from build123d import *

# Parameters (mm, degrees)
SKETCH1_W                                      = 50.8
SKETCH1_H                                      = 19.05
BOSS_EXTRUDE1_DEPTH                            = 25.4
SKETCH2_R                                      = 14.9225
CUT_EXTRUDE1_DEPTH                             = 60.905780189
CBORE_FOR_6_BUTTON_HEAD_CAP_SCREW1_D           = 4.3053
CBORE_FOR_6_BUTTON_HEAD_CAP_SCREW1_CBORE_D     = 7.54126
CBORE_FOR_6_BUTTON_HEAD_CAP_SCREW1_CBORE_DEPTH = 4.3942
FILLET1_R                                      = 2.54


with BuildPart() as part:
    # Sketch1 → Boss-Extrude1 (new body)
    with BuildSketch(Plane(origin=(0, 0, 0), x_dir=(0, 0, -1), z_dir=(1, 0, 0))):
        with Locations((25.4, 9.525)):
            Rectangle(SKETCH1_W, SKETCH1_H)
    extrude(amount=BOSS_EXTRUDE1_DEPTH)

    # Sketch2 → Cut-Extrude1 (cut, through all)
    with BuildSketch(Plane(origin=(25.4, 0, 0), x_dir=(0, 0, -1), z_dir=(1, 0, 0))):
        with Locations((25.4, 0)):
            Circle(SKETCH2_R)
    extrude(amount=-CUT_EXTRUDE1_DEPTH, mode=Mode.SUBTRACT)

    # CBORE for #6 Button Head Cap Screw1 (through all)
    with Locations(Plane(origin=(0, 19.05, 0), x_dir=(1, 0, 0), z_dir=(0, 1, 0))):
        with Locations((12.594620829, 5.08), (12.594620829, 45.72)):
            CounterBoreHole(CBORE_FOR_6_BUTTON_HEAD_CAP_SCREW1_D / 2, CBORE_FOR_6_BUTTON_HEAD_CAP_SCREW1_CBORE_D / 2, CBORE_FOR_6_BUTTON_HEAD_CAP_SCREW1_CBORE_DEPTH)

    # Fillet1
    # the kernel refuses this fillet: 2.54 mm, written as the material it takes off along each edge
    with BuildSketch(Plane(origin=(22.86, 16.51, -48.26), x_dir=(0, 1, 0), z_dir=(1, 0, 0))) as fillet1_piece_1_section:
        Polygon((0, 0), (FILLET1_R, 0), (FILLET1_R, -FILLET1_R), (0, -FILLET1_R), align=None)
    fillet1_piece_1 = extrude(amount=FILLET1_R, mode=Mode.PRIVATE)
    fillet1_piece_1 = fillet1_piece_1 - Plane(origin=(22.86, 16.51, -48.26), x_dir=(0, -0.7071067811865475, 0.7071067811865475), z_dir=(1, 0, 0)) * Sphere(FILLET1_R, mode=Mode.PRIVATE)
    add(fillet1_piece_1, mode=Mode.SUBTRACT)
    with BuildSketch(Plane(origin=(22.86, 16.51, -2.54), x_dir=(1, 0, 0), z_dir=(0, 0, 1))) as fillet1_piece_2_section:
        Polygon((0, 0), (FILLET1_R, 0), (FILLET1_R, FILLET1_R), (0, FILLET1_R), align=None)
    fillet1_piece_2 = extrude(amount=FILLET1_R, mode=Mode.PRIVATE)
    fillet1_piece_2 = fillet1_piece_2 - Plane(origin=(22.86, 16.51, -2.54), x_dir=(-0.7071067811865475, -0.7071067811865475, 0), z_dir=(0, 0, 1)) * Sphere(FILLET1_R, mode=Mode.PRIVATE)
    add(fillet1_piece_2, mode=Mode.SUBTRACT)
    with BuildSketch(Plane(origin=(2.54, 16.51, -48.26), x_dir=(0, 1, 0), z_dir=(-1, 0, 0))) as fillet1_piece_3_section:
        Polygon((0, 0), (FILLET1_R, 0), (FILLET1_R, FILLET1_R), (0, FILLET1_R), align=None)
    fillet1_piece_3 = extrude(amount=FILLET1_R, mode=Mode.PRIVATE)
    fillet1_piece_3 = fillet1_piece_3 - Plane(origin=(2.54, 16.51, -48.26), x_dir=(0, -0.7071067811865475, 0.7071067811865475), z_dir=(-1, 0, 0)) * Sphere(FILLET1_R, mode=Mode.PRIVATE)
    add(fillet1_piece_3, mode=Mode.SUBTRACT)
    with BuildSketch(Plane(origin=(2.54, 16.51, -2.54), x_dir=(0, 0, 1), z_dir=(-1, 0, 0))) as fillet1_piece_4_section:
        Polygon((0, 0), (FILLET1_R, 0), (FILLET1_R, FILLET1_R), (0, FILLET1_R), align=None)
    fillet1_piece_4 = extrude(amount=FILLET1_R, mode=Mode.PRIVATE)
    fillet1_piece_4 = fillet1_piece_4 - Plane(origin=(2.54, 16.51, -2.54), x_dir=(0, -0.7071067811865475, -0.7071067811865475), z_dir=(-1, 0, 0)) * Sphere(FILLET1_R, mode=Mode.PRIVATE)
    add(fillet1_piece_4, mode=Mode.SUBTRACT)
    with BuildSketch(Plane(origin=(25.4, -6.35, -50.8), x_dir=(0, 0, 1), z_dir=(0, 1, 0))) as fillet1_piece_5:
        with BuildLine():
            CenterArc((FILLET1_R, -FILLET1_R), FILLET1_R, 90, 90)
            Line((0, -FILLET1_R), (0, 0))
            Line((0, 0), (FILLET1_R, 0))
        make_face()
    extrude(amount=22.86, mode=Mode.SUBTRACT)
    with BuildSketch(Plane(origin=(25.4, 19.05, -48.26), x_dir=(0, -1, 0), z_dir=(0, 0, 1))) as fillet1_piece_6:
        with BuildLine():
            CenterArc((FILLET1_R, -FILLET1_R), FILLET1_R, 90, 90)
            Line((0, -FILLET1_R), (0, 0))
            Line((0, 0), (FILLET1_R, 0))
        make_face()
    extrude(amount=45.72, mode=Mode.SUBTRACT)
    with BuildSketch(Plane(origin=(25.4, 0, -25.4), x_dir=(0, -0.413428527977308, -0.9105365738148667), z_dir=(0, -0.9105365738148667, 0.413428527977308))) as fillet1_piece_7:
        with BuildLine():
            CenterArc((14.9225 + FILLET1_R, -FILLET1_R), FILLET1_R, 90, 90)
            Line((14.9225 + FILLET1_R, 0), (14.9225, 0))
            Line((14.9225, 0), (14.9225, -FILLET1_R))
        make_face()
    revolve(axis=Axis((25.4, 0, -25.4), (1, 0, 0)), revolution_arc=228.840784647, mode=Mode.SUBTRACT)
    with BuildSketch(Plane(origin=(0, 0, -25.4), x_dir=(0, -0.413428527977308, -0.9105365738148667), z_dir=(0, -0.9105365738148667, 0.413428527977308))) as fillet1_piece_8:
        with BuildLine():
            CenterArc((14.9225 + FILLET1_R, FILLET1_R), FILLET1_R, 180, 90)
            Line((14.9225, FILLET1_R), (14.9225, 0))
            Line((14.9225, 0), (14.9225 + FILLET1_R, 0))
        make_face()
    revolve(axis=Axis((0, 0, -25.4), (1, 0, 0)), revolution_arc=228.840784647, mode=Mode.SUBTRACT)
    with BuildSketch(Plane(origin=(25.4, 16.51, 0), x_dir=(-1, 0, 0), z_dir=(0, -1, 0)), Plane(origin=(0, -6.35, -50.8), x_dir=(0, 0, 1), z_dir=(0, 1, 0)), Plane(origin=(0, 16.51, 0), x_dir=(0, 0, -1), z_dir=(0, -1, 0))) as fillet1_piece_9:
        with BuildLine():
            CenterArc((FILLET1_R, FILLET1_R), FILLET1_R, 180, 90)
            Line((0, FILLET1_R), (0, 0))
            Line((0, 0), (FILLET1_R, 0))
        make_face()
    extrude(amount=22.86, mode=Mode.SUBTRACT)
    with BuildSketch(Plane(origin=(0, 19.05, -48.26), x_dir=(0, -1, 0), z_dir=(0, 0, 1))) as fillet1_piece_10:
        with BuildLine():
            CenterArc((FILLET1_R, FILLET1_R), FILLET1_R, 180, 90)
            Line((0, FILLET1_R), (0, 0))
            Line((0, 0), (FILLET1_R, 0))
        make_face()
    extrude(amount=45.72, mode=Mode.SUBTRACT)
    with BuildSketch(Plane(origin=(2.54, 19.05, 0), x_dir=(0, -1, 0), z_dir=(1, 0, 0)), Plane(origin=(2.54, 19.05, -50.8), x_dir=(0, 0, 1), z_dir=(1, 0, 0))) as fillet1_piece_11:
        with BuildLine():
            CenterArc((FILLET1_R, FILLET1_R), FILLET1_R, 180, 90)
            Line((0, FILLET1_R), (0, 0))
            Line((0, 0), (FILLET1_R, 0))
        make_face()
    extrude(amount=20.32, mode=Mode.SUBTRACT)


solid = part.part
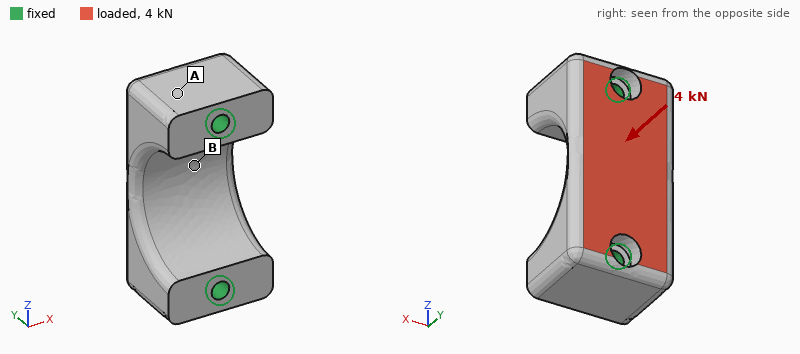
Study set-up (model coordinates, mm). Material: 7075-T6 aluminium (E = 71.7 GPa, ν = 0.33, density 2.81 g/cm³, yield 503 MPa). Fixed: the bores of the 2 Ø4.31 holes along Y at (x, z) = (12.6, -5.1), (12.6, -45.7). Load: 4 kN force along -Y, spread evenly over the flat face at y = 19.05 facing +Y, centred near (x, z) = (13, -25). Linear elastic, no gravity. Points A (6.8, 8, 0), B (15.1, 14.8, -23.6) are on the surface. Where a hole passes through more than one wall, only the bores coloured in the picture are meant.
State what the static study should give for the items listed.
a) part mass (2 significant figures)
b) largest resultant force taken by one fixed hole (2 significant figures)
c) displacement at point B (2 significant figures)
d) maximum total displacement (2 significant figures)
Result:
41 g
2.3 kN
9.7 µm
9.9 µm
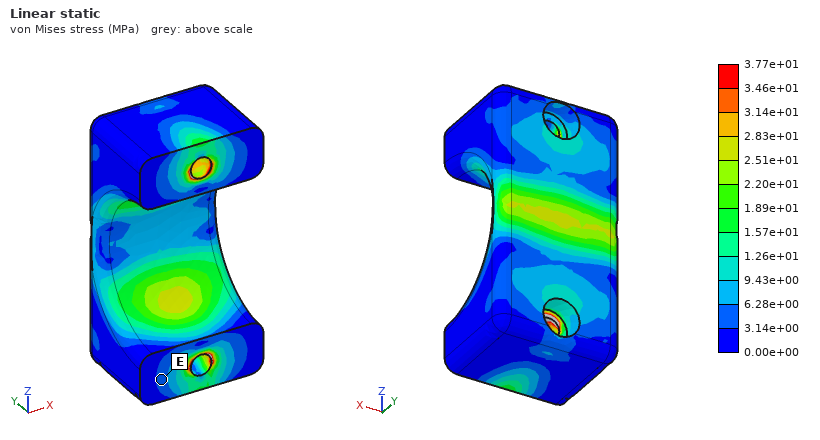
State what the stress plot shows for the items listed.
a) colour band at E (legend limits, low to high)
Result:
3.14e+00 to 6.28e+00 MPa
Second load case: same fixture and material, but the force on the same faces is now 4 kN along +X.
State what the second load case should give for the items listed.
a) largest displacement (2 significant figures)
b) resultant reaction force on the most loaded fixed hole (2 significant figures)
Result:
19 µm
2.0 kN
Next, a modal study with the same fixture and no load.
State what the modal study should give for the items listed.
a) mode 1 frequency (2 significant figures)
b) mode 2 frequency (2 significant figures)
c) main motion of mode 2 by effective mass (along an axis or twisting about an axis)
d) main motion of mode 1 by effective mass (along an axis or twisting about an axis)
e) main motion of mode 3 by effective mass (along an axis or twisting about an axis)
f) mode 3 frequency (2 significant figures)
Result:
21 kHz
29 kHz
along Y
along X
along Z
32 kHz
